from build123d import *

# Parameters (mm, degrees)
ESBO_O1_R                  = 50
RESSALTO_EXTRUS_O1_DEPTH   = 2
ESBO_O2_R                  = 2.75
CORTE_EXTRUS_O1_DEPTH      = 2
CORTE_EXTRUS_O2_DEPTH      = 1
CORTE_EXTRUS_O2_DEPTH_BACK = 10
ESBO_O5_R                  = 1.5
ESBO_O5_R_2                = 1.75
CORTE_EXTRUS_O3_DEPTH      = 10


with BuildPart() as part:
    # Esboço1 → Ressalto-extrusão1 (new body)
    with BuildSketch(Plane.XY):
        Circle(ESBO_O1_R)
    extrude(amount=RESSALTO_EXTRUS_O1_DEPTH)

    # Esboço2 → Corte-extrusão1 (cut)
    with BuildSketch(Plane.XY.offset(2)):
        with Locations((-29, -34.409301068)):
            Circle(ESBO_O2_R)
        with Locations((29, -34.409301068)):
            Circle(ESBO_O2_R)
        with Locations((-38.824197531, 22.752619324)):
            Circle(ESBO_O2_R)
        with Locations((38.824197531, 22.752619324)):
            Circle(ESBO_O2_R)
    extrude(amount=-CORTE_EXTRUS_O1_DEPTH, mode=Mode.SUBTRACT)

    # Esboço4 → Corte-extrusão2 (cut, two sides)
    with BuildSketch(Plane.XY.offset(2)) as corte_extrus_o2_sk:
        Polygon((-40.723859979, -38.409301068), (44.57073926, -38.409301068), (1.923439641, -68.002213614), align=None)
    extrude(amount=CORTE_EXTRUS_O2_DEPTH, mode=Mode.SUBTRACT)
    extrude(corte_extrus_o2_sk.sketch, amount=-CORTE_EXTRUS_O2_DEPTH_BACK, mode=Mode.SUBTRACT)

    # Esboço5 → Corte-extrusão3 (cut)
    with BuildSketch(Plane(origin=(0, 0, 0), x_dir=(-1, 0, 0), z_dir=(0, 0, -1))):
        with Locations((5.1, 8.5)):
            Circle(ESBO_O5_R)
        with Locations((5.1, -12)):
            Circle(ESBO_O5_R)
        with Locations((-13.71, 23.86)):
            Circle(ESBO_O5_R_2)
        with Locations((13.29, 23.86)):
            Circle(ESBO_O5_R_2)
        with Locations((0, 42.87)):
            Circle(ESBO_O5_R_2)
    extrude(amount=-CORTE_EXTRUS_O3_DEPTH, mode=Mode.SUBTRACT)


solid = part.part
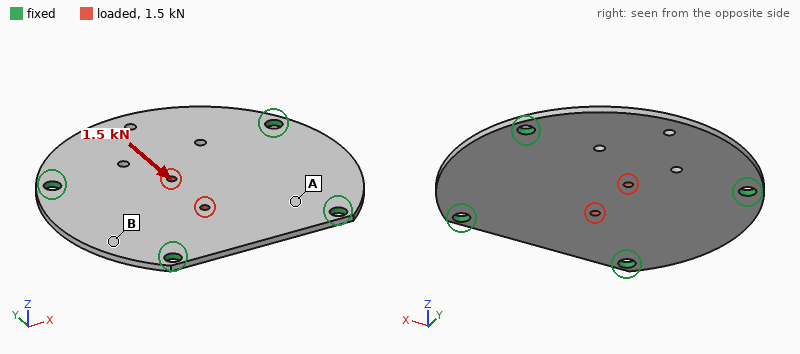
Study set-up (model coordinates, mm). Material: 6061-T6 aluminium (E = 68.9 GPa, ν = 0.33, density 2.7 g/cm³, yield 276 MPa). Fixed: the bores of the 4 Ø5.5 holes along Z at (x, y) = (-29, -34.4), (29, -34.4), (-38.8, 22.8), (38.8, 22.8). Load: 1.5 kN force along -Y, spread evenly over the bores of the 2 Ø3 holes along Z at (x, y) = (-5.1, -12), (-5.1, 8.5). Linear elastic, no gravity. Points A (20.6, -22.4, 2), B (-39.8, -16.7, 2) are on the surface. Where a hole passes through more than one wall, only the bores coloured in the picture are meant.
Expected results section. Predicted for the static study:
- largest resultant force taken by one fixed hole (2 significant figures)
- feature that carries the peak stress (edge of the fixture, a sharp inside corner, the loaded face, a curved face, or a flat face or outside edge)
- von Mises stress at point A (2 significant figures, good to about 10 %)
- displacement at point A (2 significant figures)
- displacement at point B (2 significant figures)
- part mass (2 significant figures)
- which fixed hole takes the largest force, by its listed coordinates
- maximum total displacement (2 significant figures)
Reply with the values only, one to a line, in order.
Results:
490 N
the loaded face
11 MPa
2.7 µm
2.0 µm
39 g
(-29, -34.4)
10 µm
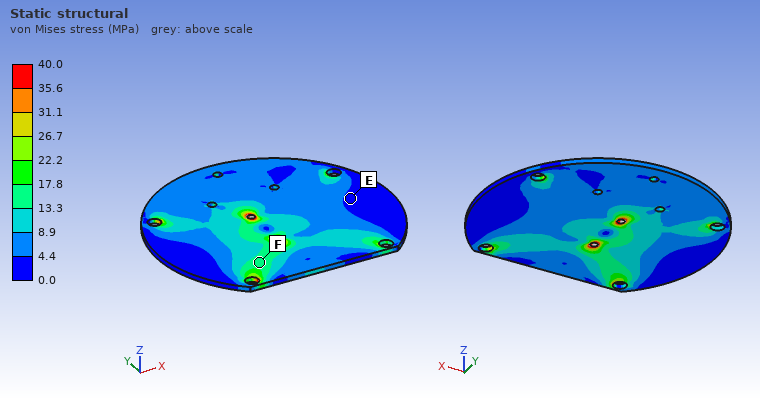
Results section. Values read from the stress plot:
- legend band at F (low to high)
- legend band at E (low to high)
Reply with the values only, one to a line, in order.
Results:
13.3 to 17.8 MPa
0.0 to 4.4 MPa
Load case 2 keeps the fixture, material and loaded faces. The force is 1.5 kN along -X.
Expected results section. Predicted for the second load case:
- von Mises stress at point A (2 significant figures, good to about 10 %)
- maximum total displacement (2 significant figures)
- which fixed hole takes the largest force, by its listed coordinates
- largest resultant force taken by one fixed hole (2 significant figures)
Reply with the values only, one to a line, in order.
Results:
8.1 MPa
8.1 µm
(-38.8, 22.8)
450 N
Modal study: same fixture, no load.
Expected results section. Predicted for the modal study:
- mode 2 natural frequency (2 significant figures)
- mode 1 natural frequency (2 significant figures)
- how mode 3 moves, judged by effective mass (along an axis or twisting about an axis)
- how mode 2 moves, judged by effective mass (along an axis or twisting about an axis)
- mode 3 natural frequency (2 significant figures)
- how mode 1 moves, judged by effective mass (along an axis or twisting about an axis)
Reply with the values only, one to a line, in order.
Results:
2000 Hz
1400 Hz
twisting about Y
along Z
3100 Hz
along Z
